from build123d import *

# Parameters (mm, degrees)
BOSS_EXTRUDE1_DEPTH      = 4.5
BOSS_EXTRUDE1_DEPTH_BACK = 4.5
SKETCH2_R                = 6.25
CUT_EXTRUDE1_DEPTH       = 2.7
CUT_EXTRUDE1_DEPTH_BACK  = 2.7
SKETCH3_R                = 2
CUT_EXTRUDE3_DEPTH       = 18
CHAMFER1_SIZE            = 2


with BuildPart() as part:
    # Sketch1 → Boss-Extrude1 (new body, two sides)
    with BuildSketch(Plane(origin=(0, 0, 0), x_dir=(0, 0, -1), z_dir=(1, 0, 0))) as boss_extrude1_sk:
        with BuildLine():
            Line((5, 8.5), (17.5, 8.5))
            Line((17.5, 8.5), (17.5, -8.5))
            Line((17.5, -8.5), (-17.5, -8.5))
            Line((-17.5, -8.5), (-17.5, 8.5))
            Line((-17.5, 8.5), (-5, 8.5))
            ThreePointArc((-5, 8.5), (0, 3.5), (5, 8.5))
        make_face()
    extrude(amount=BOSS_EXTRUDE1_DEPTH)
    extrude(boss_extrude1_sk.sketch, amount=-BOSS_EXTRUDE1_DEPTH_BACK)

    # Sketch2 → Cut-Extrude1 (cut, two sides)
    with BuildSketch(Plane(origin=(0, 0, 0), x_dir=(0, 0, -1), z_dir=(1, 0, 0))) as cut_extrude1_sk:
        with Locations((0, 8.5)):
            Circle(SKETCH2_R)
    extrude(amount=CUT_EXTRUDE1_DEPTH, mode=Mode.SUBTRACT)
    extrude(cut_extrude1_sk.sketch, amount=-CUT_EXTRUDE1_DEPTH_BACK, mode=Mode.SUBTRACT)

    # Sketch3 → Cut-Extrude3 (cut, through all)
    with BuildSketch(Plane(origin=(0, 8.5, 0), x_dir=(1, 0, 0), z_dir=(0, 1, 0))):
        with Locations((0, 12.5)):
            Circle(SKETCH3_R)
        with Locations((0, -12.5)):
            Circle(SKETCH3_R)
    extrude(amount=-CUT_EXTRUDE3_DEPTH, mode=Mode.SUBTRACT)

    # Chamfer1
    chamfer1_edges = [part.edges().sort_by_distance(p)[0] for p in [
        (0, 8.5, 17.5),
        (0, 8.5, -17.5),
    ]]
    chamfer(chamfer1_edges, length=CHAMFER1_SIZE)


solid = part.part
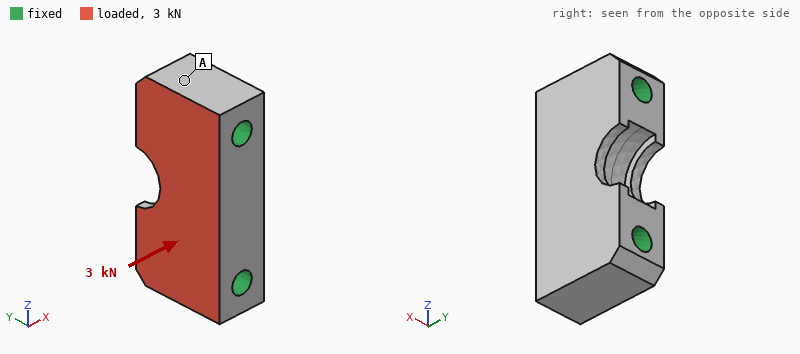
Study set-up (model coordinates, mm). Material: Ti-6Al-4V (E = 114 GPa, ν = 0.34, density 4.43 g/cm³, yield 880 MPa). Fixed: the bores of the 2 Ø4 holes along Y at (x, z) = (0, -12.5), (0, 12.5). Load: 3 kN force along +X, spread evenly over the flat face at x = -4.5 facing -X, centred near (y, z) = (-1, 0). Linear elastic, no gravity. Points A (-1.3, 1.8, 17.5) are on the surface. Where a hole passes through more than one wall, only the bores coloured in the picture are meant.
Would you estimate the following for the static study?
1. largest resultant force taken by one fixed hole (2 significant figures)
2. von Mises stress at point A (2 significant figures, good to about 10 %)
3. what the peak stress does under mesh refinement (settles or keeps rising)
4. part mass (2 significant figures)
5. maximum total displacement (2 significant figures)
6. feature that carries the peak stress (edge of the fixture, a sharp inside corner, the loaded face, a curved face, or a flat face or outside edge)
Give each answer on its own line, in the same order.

1.5 kN
3.3 MPa
keeps rising
20 g
2.2 µm
edge of the fixture
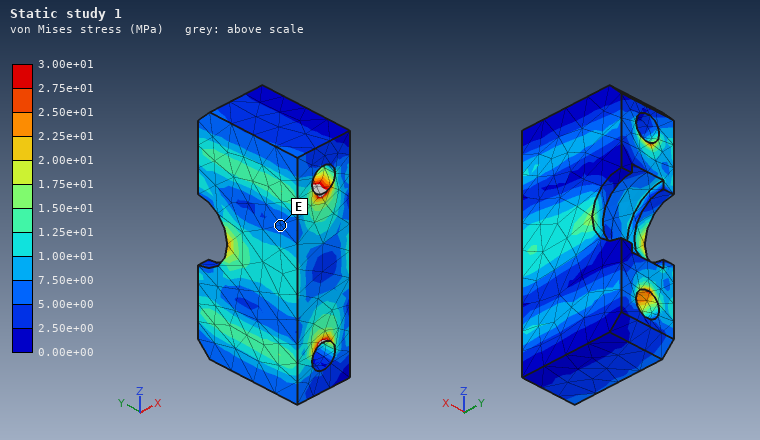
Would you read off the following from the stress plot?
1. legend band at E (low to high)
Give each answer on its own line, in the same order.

5.00e+00 to 7.50e+00 MPa
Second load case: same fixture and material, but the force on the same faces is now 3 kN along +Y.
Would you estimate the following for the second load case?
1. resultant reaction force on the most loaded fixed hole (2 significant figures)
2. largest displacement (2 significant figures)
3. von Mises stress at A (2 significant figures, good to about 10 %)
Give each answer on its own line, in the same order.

1.5 kN
3.2 µm
6.2 MPa
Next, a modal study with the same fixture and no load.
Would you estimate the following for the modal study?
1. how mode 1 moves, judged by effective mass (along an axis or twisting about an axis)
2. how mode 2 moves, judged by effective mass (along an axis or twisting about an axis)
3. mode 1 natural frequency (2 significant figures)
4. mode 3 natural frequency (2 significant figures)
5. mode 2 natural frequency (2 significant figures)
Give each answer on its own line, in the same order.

along X
along Y
48 kHz
71 kHz
65 kHz
